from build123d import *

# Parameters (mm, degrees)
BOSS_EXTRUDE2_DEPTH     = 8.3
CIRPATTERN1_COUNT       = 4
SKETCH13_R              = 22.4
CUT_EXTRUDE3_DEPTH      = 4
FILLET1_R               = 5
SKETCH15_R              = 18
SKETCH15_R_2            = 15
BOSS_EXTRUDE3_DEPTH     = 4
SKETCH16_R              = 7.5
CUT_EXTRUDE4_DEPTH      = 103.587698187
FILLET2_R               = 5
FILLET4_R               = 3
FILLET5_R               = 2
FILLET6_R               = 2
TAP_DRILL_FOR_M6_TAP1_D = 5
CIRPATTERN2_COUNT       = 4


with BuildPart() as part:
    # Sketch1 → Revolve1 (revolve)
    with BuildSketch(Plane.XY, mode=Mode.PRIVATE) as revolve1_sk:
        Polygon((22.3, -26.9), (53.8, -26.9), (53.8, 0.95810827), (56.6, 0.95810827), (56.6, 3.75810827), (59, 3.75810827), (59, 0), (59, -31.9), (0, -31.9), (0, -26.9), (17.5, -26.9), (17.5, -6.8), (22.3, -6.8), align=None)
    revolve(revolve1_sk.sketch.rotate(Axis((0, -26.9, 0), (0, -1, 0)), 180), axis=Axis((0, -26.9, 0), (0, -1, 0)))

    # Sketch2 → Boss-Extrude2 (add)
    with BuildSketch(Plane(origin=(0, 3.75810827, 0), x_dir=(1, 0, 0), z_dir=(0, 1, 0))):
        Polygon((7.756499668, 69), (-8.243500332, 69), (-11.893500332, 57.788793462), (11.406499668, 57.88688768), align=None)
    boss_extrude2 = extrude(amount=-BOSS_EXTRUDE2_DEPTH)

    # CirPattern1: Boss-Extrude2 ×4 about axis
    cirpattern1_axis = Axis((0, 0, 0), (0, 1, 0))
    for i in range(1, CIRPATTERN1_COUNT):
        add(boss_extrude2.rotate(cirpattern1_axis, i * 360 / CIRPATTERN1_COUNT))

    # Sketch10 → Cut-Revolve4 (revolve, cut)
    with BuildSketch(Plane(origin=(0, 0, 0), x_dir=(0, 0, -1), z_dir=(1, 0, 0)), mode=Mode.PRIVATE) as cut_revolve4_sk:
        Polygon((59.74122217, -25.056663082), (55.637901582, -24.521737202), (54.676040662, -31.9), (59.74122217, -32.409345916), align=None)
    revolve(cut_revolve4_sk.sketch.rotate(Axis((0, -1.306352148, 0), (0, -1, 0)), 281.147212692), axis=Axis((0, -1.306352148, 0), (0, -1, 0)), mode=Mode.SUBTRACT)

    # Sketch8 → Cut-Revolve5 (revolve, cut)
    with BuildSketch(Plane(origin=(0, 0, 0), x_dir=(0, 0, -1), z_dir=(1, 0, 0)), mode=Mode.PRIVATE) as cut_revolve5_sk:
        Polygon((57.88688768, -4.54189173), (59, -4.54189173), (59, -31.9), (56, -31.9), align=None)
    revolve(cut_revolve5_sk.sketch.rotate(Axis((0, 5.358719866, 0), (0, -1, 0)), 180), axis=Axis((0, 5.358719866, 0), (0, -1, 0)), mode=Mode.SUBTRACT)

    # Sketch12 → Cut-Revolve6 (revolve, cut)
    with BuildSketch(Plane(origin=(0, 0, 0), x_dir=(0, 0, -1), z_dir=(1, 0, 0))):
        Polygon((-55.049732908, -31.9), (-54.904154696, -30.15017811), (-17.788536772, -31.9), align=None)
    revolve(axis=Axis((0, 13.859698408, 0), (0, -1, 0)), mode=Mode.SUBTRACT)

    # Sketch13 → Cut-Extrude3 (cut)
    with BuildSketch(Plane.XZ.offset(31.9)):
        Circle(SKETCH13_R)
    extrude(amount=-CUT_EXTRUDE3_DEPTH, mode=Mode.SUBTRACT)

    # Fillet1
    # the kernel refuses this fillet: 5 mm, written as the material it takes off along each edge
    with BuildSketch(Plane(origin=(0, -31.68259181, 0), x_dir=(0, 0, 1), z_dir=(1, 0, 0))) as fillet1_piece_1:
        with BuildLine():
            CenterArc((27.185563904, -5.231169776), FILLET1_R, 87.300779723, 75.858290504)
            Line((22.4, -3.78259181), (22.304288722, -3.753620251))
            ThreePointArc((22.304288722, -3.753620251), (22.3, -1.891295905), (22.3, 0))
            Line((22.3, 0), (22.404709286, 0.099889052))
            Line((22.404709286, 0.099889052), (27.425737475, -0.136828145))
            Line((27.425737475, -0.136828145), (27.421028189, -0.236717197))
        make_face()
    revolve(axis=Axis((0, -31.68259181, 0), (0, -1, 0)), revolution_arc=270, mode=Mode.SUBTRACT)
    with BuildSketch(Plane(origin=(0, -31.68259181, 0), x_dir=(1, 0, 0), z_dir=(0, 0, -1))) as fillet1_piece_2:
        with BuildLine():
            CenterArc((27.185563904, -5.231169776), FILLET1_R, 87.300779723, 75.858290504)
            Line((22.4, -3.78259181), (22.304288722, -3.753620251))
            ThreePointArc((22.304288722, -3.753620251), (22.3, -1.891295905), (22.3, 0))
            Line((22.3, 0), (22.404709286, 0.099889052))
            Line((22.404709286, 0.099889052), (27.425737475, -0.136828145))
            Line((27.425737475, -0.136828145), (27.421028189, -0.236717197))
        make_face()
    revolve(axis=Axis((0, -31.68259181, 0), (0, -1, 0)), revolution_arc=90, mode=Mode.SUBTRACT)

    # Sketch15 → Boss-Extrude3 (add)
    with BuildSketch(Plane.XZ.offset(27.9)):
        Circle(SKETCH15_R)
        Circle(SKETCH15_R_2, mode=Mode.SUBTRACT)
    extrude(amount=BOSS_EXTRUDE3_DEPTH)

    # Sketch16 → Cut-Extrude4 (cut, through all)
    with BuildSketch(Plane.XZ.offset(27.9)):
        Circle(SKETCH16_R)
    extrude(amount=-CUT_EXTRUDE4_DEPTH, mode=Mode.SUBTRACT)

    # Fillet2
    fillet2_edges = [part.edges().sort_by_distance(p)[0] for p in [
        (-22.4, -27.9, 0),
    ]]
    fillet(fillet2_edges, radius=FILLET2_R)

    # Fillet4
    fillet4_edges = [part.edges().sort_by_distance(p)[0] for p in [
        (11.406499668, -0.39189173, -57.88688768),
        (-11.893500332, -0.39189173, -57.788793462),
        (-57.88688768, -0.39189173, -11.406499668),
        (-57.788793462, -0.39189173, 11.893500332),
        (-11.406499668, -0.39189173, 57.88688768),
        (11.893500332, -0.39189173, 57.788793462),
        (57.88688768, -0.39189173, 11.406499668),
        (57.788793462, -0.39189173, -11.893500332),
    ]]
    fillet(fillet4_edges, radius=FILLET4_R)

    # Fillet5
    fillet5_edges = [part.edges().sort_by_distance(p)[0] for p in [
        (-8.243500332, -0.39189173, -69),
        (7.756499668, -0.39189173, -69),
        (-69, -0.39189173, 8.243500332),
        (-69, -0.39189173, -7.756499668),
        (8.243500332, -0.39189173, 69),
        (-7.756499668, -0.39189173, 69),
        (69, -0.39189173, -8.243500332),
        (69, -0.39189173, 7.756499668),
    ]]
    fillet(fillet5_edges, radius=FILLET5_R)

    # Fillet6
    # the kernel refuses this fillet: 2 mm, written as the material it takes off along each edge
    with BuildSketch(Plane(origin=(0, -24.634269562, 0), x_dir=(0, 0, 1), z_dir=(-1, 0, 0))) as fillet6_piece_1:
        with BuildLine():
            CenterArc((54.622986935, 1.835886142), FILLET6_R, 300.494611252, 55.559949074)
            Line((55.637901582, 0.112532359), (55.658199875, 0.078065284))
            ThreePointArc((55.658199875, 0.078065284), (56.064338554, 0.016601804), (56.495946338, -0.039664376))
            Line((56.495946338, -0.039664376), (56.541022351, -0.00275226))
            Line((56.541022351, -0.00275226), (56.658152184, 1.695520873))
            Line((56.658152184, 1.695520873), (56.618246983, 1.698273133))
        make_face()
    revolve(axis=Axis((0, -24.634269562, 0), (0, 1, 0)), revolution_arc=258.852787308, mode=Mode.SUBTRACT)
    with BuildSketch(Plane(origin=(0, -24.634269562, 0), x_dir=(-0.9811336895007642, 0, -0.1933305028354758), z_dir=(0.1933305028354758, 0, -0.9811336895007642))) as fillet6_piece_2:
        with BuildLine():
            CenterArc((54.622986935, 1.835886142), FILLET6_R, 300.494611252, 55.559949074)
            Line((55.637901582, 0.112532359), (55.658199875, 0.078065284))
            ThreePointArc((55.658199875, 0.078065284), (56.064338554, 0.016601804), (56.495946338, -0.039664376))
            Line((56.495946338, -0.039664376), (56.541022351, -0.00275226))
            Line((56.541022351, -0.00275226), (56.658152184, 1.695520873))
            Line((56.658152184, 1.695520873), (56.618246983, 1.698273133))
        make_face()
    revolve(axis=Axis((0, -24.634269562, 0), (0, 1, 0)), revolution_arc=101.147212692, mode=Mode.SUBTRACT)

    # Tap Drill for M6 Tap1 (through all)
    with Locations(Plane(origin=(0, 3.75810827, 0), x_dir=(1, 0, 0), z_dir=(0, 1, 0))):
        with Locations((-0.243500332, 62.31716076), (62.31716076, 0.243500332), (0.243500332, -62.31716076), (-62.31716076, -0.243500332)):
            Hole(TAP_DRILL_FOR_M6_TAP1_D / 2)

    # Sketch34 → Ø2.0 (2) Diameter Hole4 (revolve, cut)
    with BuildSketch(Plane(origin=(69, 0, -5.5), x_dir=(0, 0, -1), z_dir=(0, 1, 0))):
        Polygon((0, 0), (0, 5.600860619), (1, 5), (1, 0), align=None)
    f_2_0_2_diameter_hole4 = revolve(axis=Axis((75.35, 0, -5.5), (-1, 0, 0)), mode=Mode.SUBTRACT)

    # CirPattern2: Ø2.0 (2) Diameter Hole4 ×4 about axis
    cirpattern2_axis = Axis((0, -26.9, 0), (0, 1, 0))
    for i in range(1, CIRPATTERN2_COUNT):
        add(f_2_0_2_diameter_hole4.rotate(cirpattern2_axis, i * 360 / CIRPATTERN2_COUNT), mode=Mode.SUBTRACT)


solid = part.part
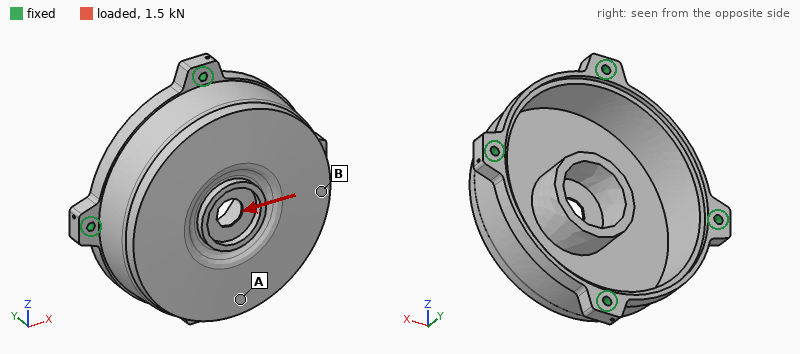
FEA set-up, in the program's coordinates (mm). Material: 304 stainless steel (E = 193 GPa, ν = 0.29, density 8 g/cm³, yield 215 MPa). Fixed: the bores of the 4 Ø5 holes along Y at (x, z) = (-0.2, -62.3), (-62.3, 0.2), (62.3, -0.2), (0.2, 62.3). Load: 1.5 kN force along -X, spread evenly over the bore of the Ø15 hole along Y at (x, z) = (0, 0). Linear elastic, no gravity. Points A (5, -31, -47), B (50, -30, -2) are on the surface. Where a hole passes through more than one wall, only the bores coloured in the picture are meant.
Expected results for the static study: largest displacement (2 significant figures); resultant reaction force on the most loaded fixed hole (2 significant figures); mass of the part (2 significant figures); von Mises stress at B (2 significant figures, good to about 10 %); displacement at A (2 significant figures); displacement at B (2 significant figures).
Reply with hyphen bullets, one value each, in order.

- 5.7 µm
- 530 N
- 710 g
- 6.6 MPa
- 2.4 µm
- 3.5 µm
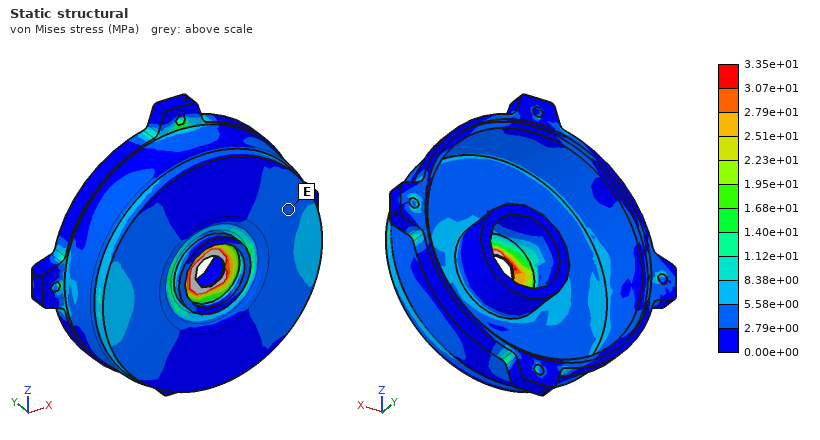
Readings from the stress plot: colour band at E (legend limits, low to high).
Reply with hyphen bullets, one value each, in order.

- 2.79e+00 to 5.58e+00 MPa
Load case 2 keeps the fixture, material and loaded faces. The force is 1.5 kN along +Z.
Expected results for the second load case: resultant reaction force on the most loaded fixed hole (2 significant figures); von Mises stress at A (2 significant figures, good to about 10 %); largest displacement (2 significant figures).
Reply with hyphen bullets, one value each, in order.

- 530 N
- 6.4 MPa
- 5.7 µm
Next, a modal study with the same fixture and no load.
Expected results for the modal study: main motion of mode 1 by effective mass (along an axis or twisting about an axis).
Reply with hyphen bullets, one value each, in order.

- along Y
